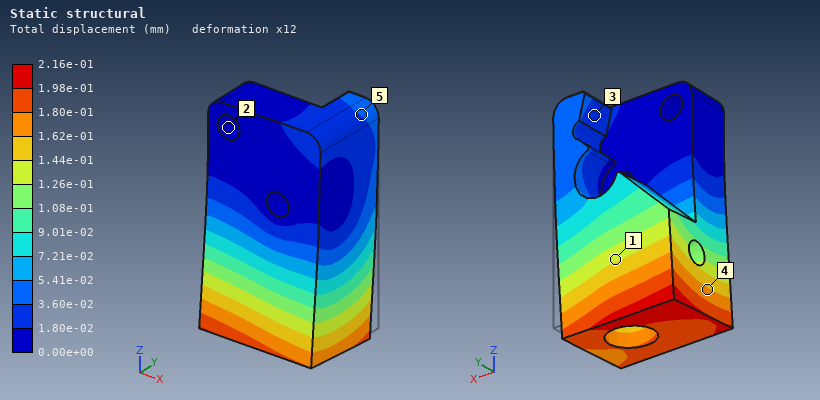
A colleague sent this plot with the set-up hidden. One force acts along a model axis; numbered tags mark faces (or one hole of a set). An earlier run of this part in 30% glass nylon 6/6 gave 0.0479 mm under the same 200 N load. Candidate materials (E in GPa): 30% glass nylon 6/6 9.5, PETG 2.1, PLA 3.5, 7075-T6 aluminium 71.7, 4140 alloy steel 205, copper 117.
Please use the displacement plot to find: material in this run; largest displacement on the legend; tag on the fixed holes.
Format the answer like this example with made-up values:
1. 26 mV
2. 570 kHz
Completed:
1. PETG
2. 2.16e-01 mm
3. 2
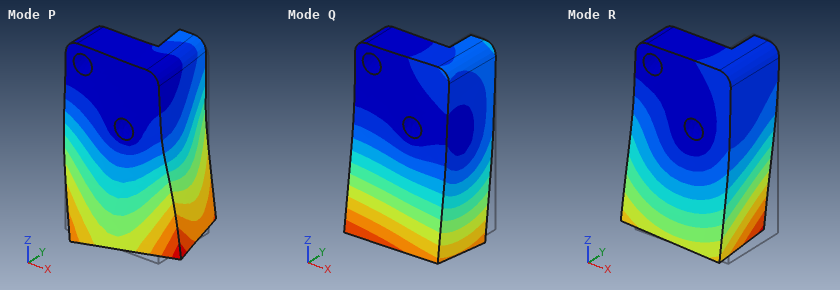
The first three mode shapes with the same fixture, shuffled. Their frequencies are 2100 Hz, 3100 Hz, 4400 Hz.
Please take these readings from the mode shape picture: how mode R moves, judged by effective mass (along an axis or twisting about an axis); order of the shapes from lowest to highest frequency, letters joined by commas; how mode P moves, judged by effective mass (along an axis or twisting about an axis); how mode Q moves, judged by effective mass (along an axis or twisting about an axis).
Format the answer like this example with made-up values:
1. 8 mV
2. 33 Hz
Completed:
1. along X
2. Q, R, P
3. twisting about Z
4. along Y
